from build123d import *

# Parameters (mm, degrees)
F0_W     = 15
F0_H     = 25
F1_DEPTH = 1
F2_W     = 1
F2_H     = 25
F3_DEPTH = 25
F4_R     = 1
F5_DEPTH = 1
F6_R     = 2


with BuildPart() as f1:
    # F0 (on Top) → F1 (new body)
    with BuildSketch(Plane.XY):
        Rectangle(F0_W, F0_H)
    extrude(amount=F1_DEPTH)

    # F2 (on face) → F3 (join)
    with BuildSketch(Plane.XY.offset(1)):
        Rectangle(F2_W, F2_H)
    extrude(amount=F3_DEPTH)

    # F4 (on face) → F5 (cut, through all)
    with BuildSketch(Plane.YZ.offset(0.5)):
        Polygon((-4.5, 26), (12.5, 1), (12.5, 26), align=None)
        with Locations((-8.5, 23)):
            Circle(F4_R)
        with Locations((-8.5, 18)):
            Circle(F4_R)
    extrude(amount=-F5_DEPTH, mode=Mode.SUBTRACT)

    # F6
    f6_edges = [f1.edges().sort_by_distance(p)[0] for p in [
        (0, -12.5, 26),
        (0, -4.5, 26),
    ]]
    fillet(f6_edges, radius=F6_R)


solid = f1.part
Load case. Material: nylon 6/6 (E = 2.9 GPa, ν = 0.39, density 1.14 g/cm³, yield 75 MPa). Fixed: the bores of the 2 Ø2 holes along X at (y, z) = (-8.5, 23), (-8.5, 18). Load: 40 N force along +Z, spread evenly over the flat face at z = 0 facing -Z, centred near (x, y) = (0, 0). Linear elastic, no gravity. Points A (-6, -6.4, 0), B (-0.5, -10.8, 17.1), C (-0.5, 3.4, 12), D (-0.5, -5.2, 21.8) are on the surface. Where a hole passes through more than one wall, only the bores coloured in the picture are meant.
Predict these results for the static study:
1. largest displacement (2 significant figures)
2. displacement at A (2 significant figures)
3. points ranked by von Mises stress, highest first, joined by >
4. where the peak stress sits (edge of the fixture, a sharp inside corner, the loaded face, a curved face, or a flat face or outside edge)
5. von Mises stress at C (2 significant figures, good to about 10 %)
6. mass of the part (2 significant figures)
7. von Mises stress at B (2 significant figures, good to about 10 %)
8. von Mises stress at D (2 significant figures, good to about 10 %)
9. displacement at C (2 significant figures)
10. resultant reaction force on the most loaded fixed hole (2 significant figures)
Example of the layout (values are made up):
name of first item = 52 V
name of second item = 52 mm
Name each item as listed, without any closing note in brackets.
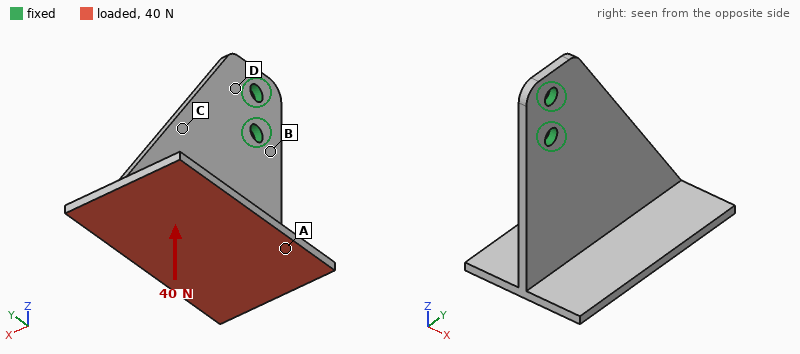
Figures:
largest displacement = 0.39 mm
displacement at A = 0.21 mm
points ranked by von Mises stress, highest first, joined by > = D > B > C > A
where the peak stress sits = edge of the fixture
von Mises stress at C = 4.5 MPa
mass of the part = 0.89 g
von Mises stress at B = 6.1 MPa
von Mises stress at D = 11 MPa
displacement at C = 0.12 mm
resultant reaction force on the most loaded fixed hole = 51 N
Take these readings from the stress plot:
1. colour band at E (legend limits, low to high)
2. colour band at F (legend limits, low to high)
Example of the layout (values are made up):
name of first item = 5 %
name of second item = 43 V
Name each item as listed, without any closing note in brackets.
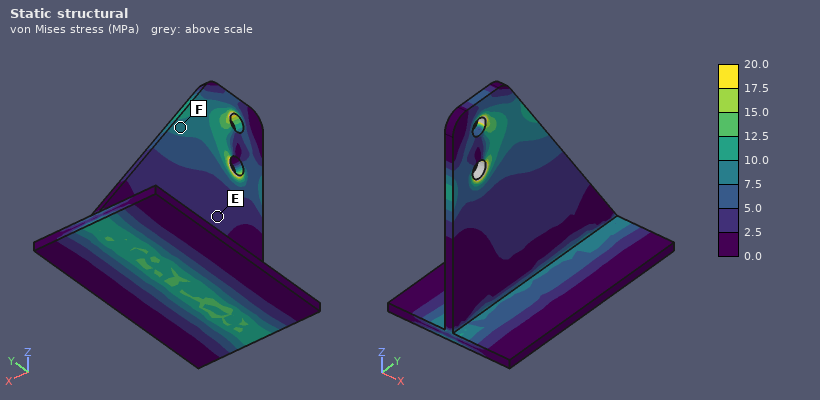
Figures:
colour band at E = 2.5 to 5.0 MPa
colour band at F = 7.5 to 10.0 MPa
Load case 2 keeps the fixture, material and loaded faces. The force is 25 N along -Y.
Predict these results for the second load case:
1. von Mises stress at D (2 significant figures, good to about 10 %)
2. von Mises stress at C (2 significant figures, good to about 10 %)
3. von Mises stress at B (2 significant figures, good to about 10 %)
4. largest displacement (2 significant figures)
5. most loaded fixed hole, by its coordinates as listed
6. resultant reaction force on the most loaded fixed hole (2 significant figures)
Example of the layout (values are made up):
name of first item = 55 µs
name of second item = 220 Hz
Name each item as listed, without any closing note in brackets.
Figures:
von Mises stress at D = 13 MPa
von Mises stress at C = 3.5 MPa
von Mises stress at B = 13 MPa
largest displacement = 0.39 mm
most loaded fixed hole, by its coordinates as listed = (-8.5, 18)
resultant reaction force on the most loaded fixed hole = 86 N
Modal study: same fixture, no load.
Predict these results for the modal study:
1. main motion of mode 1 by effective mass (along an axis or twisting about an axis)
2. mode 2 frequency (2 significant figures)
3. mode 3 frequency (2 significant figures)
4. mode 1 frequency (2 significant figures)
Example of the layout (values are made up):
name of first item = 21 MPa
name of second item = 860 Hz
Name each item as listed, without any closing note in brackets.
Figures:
main motion of mode 1 by effective mass = along X
mode 2 frequency = 560 Hz
mode 3 frequency = 1500 Hz
mode 1 frequency = 250 Hz
